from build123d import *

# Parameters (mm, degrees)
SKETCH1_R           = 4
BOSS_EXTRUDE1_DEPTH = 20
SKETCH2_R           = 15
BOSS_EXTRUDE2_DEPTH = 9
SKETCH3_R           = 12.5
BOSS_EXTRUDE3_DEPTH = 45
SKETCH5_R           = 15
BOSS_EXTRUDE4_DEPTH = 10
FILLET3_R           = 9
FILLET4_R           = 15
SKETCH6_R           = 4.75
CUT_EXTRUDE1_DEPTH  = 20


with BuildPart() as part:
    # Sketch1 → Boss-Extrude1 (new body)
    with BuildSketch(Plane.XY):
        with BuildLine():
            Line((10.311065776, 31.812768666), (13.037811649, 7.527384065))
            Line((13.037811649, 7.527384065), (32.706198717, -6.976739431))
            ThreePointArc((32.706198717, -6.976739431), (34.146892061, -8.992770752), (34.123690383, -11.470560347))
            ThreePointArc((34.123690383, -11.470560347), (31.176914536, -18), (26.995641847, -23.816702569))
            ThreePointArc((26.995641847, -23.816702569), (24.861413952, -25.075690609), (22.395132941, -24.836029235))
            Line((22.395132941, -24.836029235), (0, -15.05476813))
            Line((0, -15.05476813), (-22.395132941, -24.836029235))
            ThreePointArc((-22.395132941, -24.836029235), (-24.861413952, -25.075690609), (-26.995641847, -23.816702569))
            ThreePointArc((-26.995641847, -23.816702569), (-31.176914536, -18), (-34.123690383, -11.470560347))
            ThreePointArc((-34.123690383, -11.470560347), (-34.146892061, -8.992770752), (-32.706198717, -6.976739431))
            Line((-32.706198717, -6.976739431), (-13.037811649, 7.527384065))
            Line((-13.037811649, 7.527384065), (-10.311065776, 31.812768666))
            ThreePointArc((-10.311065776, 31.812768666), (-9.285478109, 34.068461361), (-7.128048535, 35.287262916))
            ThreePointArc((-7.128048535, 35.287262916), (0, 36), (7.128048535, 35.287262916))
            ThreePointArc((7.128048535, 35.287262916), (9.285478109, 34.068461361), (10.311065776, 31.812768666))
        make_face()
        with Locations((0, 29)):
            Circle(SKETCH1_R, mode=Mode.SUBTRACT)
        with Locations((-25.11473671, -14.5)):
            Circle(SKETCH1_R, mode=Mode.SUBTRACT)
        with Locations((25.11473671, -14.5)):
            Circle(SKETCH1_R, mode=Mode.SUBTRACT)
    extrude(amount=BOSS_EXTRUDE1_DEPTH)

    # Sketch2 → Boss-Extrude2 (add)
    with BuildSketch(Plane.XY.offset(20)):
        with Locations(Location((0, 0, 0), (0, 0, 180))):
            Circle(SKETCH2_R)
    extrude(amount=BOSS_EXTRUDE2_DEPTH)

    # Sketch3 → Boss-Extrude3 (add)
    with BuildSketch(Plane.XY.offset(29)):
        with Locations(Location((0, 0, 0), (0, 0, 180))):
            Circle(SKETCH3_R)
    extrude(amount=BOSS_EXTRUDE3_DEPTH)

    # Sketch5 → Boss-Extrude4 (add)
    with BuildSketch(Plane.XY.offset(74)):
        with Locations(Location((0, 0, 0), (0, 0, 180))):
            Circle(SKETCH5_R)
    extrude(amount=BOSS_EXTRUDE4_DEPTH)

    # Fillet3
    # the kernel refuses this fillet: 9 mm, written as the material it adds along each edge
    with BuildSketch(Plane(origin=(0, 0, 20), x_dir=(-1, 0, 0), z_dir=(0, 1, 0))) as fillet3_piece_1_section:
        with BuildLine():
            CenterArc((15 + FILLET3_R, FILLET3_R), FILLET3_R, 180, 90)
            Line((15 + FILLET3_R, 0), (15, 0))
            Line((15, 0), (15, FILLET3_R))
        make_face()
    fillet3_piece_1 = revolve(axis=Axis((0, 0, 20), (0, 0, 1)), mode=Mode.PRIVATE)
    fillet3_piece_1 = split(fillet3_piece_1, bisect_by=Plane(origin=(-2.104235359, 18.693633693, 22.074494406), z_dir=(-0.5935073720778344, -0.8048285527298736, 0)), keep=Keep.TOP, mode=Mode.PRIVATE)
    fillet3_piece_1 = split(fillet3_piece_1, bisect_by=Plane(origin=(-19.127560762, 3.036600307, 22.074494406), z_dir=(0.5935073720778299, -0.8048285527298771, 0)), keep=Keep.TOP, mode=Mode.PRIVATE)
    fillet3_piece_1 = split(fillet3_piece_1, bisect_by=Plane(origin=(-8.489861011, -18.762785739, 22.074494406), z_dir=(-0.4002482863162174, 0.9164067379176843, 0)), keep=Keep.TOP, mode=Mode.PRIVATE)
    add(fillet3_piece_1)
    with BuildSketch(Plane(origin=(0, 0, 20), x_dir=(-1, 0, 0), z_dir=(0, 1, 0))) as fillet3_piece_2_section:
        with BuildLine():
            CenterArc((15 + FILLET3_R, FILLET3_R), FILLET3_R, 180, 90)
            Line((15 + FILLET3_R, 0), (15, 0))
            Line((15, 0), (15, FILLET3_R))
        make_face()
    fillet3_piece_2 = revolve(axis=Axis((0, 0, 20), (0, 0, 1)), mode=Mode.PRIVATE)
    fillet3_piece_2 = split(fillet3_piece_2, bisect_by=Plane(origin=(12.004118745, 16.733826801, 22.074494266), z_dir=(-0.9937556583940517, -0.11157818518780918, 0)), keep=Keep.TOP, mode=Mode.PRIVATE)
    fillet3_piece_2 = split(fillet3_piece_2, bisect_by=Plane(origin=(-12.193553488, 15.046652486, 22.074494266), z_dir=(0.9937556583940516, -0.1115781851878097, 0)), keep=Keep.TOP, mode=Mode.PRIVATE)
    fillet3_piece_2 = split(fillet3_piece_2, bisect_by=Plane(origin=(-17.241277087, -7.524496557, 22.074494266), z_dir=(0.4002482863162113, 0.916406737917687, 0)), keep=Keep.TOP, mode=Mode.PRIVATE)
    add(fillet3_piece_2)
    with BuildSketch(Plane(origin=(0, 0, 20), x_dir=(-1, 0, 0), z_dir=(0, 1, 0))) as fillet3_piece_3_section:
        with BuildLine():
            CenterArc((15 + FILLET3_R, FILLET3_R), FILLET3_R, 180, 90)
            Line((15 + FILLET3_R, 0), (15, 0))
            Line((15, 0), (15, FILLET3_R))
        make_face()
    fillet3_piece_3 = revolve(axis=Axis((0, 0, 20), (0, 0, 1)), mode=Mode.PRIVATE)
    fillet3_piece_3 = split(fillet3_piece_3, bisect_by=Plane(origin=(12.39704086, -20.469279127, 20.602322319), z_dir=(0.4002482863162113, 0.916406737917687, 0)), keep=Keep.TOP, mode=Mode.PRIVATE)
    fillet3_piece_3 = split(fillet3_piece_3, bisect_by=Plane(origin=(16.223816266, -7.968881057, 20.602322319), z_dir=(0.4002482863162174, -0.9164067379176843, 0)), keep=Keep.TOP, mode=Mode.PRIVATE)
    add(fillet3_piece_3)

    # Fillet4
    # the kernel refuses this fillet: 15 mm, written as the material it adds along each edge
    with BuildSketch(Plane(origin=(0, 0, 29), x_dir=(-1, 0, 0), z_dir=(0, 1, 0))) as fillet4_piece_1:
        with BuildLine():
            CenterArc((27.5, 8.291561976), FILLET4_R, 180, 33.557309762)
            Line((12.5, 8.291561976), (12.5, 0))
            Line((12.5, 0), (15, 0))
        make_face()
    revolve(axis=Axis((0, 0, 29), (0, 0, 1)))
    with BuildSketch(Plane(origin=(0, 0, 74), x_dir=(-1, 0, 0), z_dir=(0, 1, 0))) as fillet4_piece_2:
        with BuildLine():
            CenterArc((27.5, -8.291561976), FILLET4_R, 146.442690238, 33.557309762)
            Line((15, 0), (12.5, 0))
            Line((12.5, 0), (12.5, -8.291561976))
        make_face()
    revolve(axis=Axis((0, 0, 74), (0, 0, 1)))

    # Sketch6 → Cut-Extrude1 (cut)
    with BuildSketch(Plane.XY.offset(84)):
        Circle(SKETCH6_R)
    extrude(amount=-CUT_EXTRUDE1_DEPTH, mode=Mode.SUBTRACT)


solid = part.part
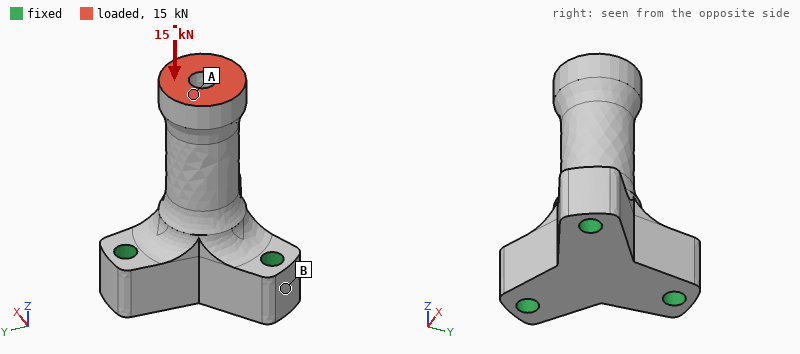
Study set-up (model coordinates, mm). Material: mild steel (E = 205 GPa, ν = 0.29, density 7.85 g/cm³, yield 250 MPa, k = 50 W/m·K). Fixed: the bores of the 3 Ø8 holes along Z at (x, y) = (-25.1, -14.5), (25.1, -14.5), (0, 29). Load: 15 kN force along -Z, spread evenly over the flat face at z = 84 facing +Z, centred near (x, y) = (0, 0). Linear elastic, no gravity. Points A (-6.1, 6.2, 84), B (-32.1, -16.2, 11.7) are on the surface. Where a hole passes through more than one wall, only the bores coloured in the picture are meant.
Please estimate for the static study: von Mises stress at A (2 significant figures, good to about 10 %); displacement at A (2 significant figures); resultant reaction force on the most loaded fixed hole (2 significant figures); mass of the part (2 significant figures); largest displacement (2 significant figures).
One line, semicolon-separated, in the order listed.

25 MPa; 12 µm; 5.3 kN; 610 g; 12 µm
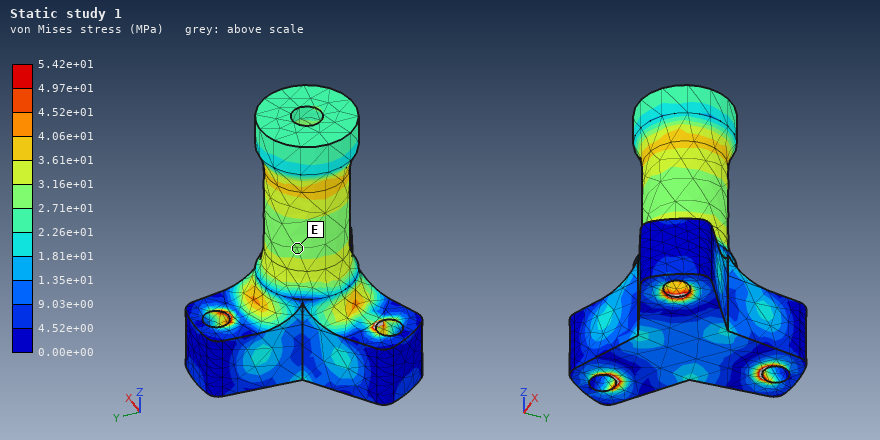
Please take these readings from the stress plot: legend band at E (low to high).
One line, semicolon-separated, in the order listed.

2.71e+01 to 3.16e+01 MPa
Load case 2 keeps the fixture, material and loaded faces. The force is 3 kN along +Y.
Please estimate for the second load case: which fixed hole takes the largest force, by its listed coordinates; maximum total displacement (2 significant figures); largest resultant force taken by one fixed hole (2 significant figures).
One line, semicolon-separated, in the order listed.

(0, 29); 69 µm; 5.5 kN
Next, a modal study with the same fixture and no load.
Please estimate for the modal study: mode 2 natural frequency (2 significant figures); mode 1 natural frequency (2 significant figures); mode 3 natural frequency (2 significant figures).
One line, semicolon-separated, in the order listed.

4000 Hz; 4000 Hz; 11 kHz
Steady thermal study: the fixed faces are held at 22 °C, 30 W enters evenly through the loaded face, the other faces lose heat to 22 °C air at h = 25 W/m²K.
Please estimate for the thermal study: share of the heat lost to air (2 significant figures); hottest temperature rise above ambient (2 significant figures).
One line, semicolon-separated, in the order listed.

21 %; 69 K
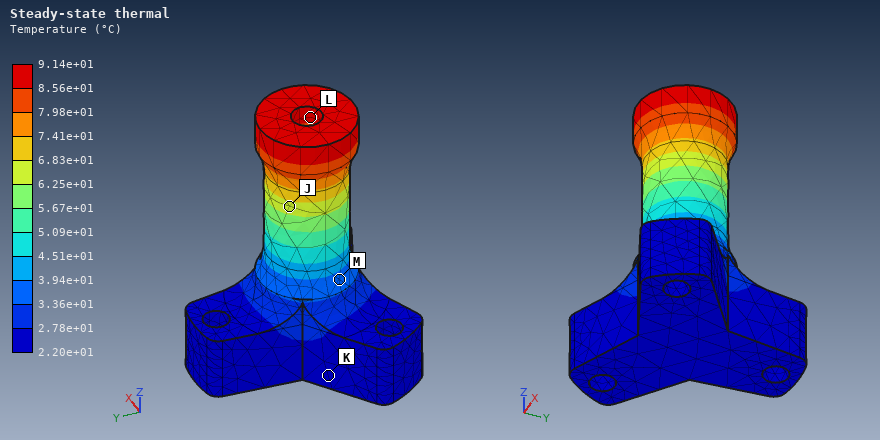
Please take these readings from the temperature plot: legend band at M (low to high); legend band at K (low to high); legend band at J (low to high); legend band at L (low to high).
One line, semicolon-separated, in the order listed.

3.36e+01 to 3.94e+01 °C; 2.20e+01 to 2.78e+01 °C; 6.25e+01 to 6.83e+01 °C; 8.56e+01 to 9.14e+01 °C
